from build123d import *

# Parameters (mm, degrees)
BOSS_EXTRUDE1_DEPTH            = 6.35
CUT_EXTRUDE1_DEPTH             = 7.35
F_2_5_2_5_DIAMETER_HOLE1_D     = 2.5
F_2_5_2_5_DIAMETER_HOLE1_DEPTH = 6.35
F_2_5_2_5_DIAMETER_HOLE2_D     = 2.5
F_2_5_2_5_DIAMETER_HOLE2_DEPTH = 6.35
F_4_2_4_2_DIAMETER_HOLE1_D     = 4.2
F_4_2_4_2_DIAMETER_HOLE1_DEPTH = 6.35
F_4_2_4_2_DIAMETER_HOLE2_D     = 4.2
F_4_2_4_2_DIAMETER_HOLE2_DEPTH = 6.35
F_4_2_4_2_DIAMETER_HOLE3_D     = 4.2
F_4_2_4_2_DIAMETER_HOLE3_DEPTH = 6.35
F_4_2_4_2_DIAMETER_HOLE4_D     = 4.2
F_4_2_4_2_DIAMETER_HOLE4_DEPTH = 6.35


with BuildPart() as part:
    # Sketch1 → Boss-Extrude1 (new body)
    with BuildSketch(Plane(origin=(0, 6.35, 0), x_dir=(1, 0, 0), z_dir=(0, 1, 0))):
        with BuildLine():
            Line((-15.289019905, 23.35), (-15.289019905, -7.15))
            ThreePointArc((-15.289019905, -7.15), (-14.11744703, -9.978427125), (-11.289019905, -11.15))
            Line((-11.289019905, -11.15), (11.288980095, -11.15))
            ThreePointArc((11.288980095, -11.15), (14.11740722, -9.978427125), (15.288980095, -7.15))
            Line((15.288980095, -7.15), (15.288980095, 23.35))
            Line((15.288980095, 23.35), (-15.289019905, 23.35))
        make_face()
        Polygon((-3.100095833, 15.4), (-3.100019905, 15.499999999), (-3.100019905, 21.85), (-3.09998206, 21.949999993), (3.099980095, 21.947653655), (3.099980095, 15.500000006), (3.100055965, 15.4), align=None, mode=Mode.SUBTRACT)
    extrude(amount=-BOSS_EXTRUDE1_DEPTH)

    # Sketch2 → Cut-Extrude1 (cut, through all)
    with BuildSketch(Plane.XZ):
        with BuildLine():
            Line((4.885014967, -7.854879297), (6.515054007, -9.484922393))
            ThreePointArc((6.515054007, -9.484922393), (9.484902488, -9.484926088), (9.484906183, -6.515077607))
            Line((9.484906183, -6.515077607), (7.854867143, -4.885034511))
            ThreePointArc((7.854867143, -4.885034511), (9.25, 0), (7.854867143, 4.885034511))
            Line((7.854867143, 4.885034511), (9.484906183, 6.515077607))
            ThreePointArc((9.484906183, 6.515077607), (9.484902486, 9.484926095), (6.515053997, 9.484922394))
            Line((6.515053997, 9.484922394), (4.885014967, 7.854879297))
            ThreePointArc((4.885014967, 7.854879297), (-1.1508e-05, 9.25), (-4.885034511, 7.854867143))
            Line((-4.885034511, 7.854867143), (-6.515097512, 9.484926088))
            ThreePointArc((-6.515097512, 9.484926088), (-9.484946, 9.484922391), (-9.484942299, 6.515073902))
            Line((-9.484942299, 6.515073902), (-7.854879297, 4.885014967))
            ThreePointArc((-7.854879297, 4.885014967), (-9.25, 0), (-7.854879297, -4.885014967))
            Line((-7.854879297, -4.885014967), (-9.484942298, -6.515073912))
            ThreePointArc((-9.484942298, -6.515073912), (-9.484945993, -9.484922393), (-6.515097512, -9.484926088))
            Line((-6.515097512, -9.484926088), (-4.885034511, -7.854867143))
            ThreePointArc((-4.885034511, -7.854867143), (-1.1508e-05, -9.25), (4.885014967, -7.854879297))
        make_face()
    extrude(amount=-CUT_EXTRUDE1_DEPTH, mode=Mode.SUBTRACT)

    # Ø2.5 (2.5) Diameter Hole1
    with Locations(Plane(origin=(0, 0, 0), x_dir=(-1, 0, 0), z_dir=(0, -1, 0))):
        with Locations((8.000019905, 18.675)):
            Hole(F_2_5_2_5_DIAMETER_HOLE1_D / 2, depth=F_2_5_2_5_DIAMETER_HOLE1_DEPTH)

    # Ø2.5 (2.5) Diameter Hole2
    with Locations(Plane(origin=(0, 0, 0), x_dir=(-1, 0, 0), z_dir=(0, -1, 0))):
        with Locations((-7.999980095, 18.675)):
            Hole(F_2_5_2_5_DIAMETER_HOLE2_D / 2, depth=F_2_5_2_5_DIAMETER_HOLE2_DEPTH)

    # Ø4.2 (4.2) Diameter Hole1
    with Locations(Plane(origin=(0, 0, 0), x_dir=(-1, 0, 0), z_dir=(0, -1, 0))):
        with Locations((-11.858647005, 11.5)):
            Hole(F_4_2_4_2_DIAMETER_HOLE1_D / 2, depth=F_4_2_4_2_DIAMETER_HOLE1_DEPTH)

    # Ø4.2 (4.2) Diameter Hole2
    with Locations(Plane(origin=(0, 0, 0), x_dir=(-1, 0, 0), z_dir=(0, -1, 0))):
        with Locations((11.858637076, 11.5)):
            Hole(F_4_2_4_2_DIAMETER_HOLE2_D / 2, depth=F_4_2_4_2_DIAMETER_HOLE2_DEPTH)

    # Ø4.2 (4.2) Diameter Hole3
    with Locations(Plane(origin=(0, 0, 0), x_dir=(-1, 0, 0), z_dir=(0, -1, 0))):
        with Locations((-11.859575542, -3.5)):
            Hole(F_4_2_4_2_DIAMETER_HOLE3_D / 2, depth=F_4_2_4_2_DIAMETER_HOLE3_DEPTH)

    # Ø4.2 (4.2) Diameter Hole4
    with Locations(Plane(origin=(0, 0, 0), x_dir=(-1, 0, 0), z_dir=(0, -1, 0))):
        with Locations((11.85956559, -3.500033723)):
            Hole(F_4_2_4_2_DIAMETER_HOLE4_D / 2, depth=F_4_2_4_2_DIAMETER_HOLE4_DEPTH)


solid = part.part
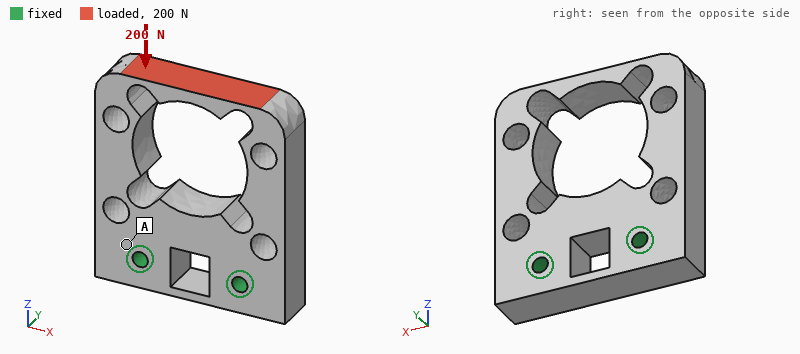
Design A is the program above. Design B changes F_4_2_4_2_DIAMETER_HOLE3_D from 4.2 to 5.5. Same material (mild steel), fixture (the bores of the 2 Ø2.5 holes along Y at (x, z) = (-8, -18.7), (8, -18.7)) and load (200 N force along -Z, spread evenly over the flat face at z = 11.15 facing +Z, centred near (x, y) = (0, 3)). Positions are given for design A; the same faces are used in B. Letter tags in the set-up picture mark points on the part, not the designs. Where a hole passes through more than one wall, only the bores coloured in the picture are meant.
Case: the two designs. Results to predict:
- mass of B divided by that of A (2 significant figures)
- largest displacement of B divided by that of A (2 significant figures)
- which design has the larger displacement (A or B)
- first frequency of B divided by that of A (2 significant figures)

0.98
1.1
B
1.0
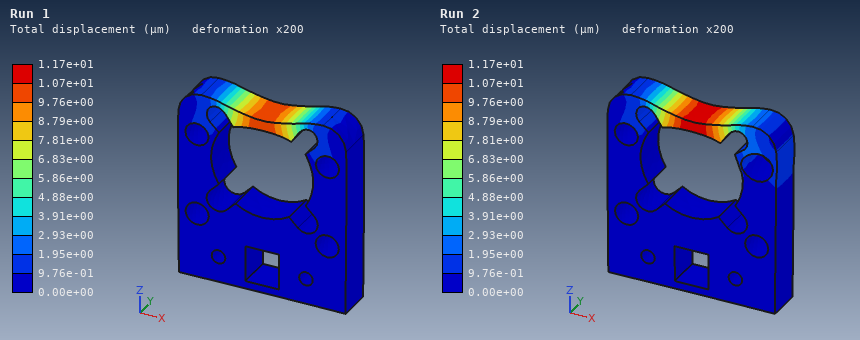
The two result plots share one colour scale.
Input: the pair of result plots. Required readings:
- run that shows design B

Run 2
